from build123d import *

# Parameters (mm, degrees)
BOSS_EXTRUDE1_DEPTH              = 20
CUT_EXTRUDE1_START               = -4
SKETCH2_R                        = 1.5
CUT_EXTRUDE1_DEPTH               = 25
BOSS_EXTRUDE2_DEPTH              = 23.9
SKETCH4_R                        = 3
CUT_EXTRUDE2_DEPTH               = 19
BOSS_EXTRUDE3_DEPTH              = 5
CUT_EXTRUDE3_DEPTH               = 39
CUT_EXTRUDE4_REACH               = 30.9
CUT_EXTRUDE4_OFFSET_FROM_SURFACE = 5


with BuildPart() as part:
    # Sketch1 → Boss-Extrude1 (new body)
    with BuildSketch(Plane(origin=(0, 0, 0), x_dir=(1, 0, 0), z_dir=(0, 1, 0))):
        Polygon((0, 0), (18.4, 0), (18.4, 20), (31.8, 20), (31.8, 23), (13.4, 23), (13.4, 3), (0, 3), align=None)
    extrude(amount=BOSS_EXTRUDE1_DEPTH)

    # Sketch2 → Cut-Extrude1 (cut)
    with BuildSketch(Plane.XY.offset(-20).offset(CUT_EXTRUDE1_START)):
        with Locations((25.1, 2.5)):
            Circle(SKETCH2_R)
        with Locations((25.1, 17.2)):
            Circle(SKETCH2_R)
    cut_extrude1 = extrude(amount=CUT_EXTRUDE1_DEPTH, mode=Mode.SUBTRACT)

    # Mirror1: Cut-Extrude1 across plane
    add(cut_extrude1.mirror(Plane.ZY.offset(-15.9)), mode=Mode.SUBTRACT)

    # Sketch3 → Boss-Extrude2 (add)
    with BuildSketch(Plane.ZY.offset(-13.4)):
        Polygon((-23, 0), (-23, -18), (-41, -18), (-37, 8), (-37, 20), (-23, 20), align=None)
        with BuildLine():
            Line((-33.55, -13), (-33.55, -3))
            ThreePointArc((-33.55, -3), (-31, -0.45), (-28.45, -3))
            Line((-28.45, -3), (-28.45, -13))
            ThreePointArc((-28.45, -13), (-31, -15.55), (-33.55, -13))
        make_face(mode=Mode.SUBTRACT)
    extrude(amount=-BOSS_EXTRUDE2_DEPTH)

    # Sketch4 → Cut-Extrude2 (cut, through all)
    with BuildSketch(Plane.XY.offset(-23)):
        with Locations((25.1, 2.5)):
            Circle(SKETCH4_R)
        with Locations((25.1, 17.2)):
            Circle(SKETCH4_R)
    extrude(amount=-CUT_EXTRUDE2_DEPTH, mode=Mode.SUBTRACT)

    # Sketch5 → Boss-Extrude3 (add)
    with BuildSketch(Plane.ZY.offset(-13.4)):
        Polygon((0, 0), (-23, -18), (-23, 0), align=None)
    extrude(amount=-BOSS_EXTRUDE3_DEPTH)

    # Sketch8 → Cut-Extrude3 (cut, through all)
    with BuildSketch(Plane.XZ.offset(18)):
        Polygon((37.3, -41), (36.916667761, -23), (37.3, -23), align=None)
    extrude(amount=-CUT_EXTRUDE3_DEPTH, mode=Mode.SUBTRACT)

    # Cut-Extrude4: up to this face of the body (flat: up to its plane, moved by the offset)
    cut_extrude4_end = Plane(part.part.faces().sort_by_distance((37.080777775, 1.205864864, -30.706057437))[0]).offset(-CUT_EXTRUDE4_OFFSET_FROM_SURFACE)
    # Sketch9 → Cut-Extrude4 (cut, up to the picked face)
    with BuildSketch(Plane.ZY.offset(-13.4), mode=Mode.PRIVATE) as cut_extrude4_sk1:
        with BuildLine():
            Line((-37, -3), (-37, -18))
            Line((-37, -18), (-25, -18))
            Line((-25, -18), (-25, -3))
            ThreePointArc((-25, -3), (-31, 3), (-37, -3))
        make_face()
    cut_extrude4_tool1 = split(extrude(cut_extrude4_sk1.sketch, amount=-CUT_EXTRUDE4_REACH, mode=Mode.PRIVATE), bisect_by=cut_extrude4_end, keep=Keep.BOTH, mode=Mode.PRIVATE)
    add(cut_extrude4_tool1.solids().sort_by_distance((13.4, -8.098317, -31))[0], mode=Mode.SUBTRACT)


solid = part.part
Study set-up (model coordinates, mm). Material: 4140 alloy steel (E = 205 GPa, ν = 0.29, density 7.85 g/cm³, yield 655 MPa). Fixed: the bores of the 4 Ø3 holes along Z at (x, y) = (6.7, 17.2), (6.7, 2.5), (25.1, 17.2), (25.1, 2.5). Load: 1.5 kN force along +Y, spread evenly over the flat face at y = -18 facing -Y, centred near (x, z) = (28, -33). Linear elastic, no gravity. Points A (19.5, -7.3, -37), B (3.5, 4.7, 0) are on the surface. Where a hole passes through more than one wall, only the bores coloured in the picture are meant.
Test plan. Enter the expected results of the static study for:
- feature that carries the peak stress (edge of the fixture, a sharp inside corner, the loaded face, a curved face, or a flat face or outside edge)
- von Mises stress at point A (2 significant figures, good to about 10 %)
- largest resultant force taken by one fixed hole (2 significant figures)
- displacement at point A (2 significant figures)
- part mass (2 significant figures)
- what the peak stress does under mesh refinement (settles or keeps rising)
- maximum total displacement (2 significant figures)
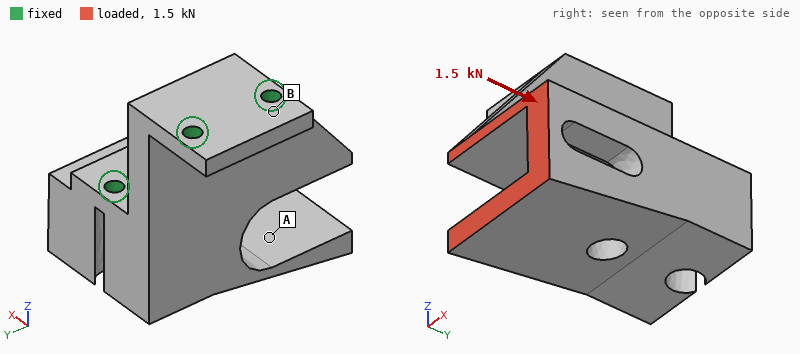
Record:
edge of the fixture
20 MPa
1.2 kN
10 µm
100 g
keeps rising
22 µm
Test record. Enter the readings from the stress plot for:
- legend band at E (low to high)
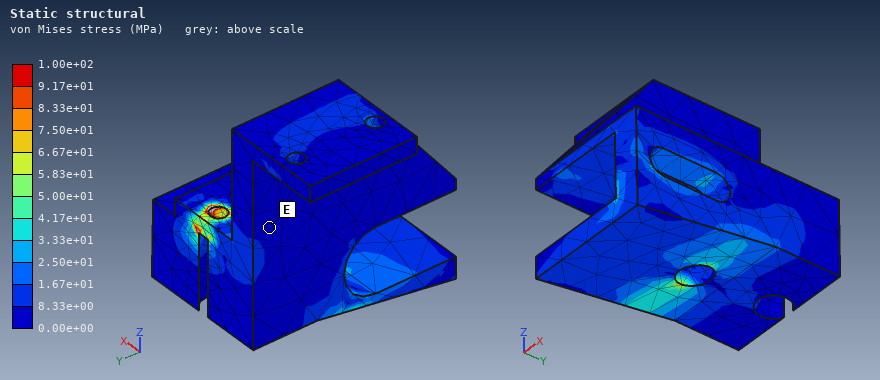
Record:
0.00e+00 to 8.33e+00 MPa
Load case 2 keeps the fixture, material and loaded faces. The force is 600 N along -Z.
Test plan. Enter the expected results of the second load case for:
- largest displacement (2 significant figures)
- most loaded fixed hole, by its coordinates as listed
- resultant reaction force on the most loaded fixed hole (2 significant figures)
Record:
64 µm
(25.1, 2.5)
1.1 kN
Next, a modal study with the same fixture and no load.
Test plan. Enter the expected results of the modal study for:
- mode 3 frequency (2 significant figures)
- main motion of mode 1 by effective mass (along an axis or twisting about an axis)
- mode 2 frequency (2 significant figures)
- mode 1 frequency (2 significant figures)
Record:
11 kHz
along X
6400 Hz
6100 Hz
